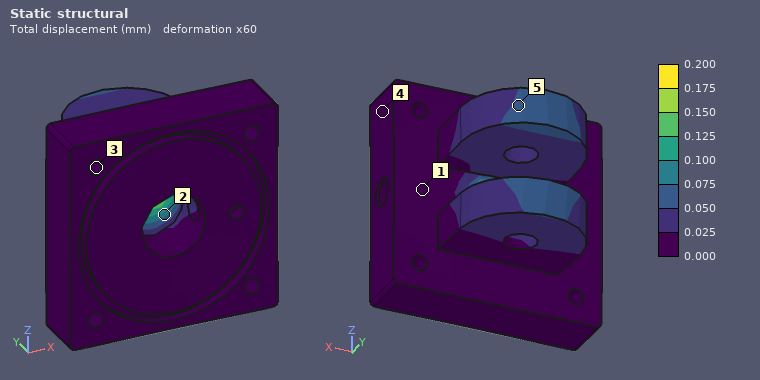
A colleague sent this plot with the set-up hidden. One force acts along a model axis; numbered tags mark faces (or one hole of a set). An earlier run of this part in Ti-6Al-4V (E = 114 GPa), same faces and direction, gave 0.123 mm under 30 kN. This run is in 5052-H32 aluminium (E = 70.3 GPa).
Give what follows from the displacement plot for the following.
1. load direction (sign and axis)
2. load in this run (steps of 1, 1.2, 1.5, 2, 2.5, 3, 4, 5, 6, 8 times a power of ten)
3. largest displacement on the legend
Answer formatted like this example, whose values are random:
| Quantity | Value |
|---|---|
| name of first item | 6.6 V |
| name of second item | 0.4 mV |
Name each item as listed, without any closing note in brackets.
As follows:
| Quantity | Value |
|---|---|
| load direction | +Y |
| load in this run | 30 kN |
| largest displacement on the legend | 0.200 mm |
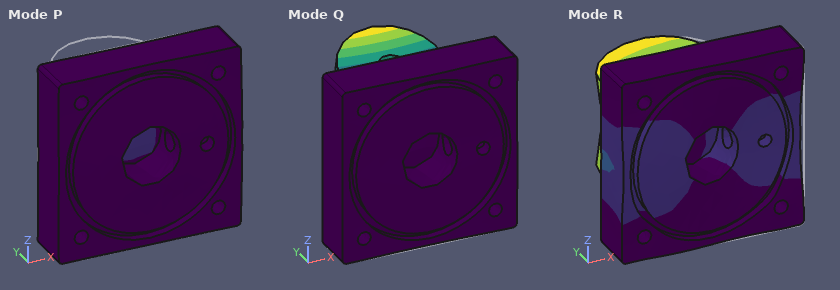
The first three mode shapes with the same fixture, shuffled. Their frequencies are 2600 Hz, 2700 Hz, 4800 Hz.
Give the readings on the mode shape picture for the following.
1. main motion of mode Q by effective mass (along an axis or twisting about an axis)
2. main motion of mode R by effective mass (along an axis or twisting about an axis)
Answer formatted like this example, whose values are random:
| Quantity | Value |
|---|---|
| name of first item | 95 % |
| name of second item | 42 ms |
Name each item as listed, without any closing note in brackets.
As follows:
| Quantity | Value |
|---|---|
| main motion of mode Q by effective mass | along Z |
| main motion of mode R by effective mass | along X |
